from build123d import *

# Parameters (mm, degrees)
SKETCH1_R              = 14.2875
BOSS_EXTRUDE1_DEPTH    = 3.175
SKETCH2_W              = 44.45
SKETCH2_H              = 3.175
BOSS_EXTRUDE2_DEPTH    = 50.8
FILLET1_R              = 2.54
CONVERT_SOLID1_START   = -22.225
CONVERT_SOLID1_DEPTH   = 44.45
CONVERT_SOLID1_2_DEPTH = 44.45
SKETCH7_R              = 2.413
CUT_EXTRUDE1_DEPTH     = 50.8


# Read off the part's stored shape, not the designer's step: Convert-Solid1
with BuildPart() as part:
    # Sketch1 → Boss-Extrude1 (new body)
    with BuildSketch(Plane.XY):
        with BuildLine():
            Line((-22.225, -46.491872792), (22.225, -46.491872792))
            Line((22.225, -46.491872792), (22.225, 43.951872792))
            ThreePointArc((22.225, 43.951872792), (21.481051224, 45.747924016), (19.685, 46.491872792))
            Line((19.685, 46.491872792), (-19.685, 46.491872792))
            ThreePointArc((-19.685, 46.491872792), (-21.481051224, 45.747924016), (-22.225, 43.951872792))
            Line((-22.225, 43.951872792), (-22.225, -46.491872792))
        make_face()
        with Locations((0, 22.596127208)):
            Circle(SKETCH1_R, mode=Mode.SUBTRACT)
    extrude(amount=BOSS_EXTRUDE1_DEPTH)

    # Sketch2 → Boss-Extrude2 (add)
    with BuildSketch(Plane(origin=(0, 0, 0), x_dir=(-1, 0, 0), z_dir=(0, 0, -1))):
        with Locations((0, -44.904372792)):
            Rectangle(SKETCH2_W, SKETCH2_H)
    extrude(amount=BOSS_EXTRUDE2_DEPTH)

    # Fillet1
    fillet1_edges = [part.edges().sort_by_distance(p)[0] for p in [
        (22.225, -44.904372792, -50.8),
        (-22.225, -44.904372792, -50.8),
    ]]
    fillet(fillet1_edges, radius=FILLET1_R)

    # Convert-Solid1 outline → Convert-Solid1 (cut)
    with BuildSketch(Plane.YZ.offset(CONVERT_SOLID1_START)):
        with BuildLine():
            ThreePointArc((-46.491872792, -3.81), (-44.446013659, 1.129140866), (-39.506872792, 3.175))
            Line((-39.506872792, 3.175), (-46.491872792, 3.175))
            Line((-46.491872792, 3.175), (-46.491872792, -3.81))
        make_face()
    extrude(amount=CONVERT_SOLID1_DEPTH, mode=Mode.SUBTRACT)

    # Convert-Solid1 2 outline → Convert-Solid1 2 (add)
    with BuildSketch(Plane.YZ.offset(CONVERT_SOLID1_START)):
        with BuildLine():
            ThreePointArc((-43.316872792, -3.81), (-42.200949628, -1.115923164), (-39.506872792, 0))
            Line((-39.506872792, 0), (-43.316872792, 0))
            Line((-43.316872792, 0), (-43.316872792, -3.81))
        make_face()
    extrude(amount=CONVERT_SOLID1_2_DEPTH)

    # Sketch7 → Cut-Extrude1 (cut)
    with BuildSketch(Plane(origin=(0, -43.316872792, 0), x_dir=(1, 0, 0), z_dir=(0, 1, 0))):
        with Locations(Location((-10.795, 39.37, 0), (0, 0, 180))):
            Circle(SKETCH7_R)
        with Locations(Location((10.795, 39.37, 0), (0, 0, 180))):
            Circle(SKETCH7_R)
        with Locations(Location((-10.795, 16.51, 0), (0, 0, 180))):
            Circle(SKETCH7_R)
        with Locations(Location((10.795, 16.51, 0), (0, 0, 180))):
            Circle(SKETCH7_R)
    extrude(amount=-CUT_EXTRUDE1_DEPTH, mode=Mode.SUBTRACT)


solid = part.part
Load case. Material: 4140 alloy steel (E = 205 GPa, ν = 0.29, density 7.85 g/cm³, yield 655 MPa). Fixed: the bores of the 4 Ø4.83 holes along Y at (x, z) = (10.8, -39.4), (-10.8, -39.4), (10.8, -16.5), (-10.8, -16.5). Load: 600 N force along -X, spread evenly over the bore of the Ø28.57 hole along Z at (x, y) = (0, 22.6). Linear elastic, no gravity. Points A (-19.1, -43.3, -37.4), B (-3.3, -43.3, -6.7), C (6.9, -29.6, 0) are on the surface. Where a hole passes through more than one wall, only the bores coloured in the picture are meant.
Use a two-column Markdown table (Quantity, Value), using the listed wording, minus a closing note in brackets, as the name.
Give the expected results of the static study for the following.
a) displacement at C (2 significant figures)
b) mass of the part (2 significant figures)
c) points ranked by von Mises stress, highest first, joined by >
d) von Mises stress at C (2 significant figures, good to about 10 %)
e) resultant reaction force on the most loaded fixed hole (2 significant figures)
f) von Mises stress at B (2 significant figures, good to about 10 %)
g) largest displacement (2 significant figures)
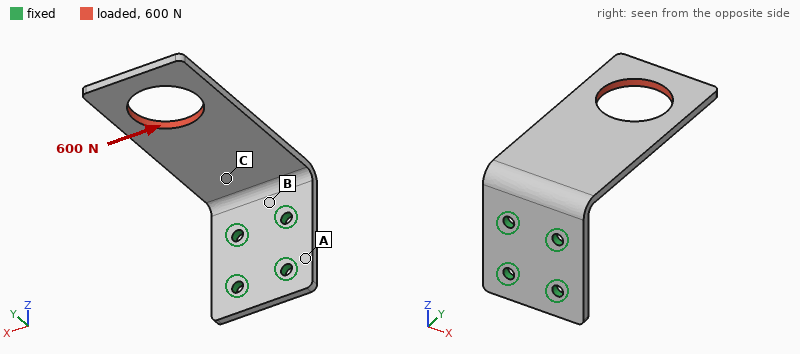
| Quantity | Value |
|---|---|
| displacement at C | 0.12 mm |
| mass of the part | 140 g |
| points ranked by von Mises stress, highest first, joined by > | B > C > A |
| von Mises stress at C | 68 MPa |
| resultant reaction force on the most loaded fixed hole | 1.6 kN |
| von Mises stress at B | 230 MPa |
| largest displacement | 0.70 mm |
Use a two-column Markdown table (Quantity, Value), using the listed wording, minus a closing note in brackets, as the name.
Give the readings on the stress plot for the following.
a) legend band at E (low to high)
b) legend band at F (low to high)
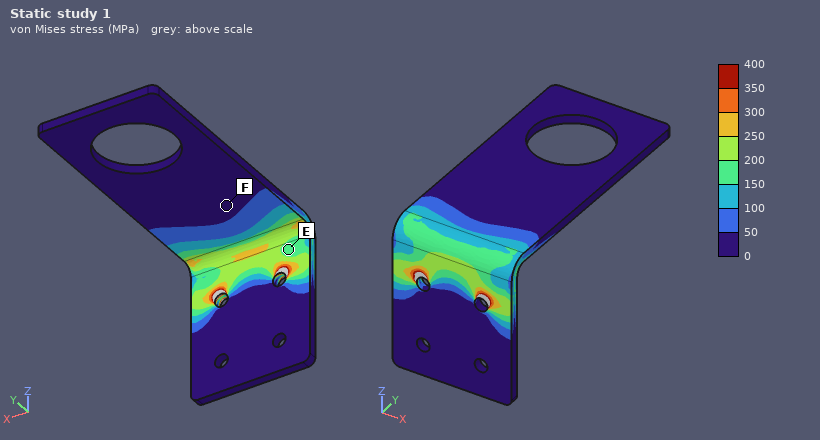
| Quantity | Value |
|---|---|
| legend band at E | 150 to 200 MPa |
| legend band at F | 0 to 50 MPa |
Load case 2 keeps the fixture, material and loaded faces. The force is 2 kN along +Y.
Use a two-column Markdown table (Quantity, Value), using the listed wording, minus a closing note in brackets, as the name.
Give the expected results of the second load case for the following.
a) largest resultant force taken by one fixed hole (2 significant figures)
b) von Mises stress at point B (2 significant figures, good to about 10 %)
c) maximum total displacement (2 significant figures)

| Quantity | Value |
|---|---|
| largest resultant force taken by one fixed hole | 1.1 kN |
| von Mises stress at point B | 210 MPa |
| maximum total displacement | 1.1 mm |
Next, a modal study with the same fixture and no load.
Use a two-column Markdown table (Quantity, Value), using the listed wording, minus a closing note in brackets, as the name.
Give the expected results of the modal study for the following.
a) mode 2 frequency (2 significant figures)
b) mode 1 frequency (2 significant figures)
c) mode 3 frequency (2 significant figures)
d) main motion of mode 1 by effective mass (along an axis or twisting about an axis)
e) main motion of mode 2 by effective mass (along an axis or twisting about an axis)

| Quantity | Value |
|---|---|
| mode 2 frequency | 780 Hz |
| mode 1 frequency | 290 Hz |
| mode 3 frequency | 1300 Hz |
| main motion of mode 1 by effective mass | along Z |
| main motion of mode 2 by effective mass | along X |
